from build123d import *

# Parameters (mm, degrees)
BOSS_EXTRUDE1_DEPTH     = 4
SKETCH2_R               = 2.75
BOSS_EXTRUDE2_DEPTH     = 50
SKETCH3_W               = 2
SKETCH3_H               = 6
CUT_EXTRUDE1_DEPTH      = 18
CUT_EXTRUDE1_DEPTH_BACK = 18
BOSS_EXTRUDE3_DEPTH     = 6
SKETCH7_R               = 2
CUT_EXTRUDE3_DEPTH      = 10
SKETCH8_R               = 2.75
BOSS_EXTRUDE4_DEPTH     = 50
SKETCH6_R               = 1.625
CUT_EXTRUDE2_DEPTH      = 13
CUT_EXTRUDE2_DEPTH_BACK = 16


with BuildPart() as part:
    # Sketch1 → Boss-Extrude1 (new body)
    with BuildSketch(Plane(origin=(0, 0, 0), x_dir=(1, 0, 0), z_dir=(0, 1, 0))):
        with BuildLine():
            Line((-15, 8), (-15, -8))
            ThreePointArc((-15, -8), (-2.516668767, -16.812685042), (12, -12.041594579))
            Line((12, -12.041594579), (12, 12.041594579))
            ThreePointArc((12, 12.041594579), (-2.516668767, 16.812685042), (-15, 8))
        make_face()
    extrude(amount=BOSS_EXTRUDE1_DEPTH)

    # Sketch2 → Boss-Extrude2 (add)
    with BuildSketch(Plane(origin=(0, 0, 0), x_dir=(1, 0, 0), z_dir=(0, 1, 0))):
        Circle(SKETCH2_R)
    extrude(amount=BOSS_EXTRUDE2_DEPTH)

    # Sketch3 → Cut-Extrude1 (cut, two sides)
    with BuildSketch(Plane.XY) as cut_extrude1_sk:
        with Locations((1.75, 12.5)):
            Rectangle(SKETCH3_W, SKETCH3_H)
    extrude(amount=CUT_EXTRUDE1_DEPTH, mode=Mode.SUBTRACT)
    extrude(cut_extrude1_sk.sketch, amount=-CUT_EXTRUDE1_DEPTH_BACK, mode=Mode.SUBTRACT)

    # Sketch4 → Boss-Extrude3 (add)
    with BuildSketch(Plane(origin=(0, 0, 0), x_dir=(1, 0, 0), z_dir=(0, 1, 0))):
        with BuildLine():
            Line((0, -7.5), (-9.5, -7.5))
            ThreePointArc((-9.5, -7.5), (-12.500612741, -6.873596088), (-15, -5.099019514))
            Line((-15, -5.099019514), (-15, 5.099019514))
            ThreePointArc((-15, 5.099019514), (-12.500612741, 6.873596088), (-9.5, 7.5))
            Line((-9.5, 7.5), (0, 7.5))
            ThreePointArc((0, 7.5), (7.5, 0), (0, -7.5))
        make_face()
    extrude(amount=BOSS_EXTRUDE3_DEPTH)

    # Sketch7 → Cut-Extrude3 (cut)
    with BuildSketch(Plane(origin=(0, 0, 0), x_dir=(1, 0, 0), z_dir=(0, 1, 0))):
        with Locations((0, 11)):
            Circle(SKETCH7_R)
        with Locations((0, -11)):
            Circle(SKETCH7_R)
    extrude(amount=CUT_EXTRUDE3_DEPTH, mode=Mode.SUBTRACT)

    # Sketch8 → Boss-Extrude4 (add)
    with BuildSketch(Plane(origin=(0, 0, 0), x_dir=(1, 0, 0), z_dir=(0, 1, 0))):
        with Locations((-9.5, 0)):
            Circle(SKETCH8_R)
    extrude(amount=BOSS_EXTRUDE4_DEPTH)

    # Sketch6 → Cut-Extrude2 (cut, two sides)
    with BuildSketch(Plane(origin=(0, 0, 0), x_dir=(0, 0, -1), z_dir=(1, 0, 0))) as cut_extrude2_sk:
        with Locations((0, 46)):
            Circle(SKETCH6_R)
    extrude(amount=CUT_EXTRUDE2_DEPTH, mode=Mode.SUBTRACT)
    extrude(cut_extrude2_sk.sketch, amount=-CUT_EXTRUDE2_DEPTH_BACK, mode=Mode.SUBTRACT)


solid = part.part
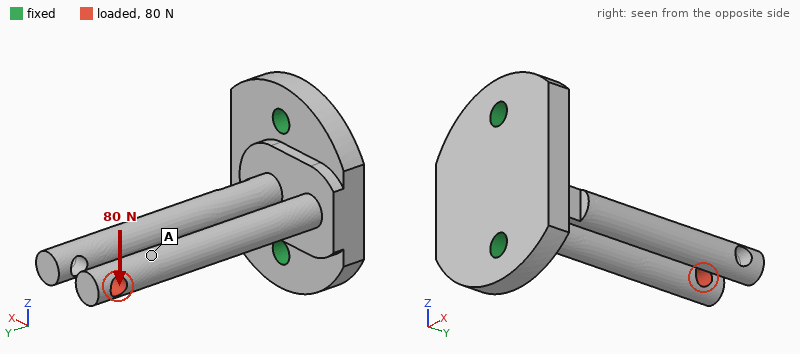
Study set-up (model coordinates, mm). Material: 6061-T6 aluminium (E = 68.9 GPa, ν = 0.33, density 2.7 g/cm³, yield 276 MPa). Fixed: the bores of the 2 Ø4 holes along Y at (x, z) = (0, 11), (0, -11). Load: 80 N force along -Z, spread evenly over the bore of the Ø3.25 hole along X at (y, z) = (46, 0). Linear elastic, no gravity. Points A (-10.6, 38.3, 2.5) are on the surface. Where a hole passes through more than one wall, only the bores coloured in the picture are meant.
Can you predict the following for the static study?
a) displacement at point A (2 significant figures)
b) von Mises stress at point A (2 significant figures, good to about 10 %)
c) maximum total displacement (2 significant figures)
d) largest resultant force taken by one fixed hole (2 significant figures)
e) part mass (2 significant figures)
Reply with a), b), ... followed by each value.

a) 0.46 mm
b) 35 MPa
c) 0.73 mm
d) 190 N
e) 15 g
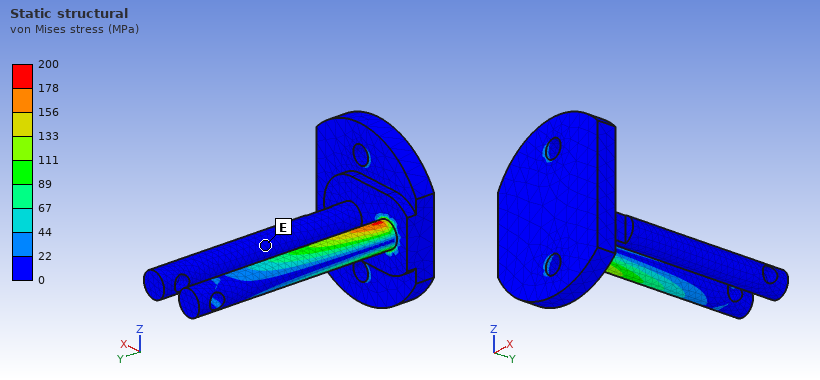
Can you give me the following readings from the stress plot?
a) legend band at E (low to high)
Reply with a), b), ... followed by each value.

a) 0 to 22 MPa
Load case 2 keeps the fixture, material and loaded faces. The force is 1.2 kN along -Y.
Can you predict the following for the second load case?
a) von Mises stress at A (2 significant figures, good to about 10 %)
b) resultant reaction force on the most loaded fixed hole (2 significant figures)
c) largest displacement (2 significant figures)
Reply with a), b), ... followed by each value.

a) 51 MPa
b) 680 N
c) 0.20 mm
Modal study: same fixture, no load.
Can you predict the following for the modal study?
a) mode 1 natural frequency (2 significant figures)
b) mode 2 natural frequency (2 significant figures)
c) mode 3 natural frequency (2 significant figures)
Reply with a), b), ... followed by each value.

a) 1400 Hz
b) 1800 Hz
c) 1900 Hz
